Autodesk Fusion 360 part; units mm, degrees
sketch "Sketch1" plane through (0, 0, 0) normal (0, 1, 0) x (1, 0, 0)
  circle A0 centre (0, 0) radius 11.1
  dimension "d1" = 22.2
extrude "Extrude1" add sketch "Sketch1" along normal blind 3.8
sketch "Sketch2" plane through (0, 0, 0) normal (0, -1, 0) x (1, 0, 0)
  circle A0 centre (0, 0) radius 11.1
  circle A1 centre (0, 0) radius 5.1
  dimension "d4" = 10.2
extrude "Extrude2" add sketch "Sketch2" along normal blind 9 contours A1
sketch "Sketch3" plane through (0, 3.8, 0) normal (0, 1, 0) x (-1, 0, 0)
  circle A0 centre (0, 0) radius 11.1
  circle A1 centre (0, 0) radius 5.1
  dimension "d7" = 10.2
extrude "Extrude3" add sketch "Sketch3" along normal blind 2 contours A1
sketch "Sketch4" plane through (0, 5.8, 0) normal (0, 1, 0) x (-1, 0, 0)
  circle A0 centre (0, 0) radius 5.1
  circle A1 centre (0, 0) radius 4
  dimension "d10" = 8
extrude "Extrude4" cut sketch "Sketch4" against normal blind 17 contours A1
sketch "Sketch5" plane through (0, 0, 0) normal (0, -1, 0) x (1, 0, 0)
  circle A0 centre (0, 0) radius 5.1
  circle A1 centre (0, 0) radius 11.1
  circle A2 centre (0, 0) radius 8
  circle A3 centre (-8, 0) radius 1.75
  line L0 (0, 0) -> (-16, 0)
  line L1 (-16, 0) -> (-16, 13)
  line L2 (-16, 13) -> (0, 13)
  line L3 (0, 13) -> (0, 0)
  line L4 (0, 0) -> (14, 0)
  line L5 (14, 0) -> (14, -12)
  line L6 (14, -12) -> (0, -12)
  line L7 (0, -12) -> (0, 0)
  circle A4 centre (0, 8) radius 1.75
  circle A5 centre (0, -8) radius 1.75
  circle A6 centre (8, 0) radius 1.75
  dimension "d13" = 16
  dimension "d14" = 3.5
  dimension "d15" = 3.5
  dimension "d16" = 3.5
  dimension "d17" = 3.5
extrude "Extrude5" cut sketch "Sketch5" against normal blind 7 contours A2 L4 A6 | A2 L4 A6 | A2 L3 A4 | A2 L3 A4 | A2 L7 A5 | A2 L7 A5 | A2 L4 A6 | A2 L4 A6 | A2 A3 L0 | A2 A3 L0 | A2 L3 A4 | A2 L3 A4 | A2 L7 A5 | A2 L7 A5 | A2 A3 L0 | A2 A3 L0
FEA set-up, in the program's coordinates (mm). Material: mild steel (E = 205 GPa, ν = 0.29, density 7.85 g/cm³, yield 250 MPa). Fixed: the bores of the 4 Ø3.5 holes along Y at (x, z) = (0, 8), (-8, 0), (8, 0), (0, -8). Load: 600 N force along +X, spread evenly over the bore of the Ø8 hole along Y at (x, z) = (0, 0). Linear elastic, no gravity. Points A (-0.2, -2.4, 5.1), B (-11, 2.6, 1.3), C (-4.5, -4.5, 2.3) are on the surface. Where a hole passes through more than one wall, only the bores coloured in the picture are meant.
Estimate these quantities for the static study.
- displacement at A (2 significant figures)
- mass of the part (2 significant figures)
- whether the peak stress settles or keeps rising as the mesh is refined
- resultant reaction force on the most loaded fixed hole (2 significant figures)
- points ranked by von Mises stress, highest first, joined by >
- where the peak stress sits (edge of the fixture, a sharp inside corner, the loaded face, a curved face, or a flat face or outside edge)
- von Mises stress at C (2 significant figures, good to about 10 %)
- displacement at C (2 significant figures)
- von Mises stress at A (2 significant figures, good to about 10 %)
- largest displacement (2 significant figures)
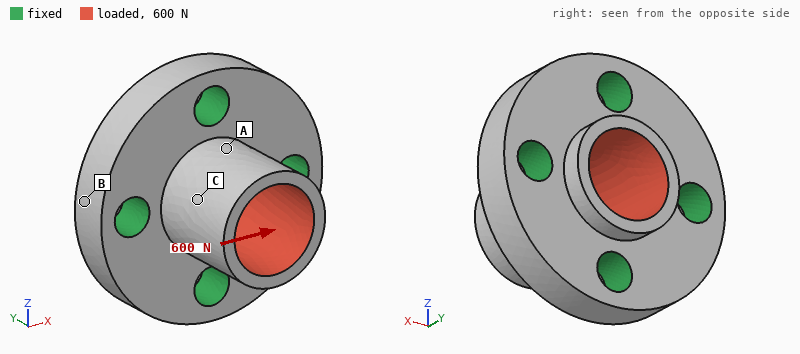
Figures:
0.90 µm
12 g
keeps rising
220 N
A > C > B
a sharp inside corner
11 MPa
1.7 µm
22 MPa
2.7 µm
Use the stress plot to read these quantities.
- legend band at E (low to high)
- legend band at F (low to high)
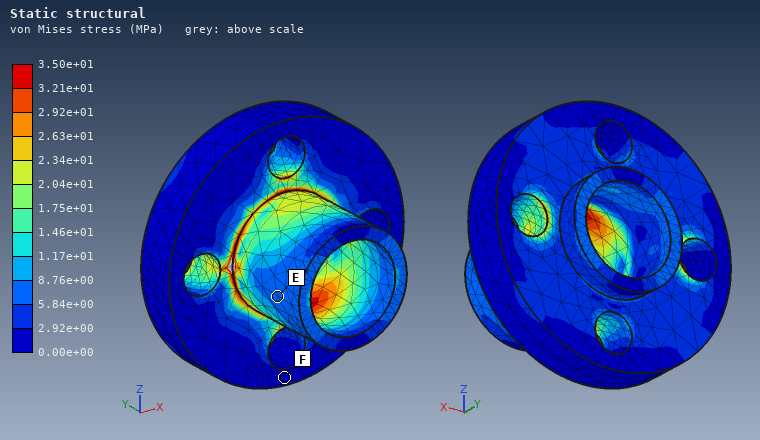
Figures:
5.84e+00 to 8.76e+00 MPa
0.00e+00 to 2.92e+00 MPa
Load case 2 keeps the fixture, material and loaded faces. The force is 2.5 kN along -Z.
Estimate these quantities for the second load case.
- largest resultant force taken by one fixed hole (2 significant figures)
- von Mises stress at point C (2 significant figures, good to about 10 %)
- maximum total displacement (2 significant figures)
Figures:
930 N
69 MPa
11 µm
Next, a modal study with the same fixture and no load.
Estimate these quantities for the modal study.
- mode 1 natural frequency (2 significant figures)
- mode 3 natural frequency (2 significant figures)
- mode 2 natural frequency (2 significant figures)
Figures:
45 kHz
46 kHz
46 kHz
